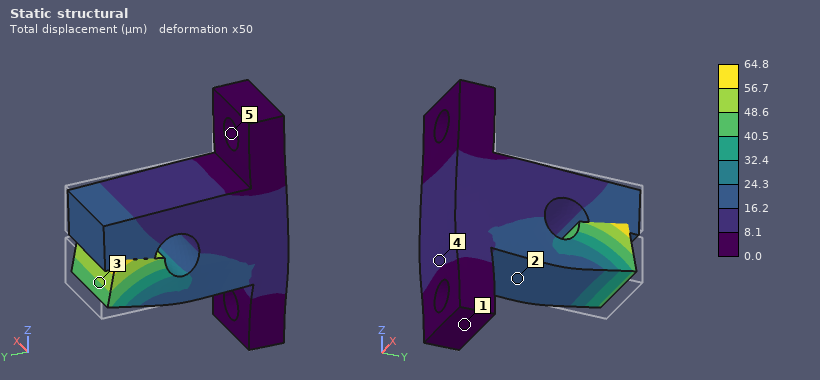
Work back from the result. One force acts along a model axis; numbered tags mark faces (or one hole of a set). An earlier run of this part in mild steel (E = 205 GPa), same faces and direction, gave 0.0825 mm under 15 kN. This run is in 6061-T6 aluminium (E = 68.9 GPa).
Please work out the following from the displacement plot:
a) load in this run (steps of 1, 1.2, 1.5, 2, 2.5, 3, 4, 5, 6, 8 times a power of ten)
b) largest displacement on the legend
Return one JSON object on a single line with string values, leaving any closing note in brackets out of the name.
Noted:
{"load in this run": "4 kN", "largest displacement on the legend": "64.8 µm"}
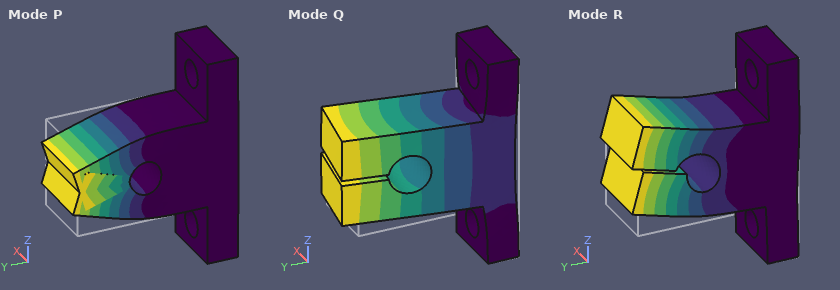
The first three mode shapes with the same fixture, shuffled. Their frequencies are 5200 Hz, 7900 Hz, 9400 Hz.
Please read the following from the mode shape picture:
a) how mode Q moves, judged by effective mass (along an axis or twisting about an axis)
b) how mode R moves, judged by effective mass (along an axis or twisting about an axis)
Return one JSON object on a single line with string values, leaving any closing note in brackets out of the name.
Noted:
{"how mode Q moves, judged by effective mass": "along X", "how mode R moves, judged by effective mass": "along Z"}
